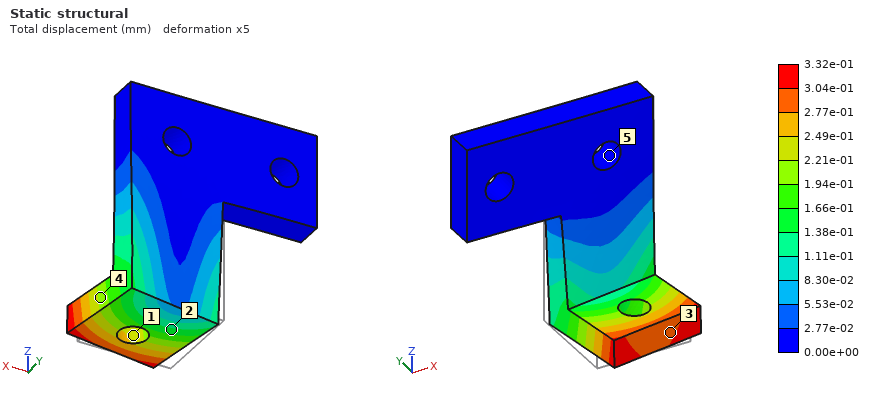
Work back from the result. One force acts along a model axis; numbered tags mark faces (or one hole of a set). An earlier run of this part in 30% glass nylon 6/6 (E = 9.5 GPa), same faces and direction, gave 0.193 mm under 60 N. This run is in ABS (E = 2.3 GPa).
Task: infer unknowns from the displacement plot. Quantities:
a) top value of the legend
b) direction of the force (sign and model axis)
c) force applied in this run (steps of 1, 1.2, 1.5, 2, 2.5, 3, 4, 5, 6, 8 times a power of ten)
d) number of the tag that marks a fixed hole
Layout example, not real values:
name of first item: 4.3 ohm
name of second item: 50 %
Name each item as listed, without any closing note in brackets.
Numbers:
top value of the legend: 3.32e-01 mm
direction of the force: +X
force applied in this run: 25 N
number of the tag that marks a fixed hole: 5
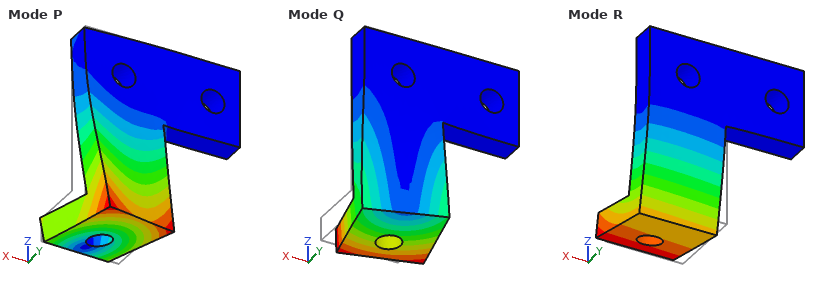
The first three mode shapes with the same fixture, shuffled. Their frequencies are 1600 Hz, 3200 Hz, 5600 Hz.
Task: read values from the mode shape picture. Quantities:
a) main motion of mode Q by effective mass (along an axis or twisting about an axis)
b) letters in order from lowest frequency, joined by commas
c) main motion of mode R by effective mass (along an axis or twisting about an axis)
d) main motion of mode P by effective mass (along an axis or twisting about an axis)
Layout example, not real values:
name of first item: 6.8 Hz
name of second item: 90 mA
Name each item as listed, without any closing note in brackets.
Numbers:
main motion of mode Q by effective mass: along X
letters in order from lowest frequency, joined by commas: R, Q, P
main motion of mode R by effective mass: along Y
main motion of mode P by effective mass: along X
